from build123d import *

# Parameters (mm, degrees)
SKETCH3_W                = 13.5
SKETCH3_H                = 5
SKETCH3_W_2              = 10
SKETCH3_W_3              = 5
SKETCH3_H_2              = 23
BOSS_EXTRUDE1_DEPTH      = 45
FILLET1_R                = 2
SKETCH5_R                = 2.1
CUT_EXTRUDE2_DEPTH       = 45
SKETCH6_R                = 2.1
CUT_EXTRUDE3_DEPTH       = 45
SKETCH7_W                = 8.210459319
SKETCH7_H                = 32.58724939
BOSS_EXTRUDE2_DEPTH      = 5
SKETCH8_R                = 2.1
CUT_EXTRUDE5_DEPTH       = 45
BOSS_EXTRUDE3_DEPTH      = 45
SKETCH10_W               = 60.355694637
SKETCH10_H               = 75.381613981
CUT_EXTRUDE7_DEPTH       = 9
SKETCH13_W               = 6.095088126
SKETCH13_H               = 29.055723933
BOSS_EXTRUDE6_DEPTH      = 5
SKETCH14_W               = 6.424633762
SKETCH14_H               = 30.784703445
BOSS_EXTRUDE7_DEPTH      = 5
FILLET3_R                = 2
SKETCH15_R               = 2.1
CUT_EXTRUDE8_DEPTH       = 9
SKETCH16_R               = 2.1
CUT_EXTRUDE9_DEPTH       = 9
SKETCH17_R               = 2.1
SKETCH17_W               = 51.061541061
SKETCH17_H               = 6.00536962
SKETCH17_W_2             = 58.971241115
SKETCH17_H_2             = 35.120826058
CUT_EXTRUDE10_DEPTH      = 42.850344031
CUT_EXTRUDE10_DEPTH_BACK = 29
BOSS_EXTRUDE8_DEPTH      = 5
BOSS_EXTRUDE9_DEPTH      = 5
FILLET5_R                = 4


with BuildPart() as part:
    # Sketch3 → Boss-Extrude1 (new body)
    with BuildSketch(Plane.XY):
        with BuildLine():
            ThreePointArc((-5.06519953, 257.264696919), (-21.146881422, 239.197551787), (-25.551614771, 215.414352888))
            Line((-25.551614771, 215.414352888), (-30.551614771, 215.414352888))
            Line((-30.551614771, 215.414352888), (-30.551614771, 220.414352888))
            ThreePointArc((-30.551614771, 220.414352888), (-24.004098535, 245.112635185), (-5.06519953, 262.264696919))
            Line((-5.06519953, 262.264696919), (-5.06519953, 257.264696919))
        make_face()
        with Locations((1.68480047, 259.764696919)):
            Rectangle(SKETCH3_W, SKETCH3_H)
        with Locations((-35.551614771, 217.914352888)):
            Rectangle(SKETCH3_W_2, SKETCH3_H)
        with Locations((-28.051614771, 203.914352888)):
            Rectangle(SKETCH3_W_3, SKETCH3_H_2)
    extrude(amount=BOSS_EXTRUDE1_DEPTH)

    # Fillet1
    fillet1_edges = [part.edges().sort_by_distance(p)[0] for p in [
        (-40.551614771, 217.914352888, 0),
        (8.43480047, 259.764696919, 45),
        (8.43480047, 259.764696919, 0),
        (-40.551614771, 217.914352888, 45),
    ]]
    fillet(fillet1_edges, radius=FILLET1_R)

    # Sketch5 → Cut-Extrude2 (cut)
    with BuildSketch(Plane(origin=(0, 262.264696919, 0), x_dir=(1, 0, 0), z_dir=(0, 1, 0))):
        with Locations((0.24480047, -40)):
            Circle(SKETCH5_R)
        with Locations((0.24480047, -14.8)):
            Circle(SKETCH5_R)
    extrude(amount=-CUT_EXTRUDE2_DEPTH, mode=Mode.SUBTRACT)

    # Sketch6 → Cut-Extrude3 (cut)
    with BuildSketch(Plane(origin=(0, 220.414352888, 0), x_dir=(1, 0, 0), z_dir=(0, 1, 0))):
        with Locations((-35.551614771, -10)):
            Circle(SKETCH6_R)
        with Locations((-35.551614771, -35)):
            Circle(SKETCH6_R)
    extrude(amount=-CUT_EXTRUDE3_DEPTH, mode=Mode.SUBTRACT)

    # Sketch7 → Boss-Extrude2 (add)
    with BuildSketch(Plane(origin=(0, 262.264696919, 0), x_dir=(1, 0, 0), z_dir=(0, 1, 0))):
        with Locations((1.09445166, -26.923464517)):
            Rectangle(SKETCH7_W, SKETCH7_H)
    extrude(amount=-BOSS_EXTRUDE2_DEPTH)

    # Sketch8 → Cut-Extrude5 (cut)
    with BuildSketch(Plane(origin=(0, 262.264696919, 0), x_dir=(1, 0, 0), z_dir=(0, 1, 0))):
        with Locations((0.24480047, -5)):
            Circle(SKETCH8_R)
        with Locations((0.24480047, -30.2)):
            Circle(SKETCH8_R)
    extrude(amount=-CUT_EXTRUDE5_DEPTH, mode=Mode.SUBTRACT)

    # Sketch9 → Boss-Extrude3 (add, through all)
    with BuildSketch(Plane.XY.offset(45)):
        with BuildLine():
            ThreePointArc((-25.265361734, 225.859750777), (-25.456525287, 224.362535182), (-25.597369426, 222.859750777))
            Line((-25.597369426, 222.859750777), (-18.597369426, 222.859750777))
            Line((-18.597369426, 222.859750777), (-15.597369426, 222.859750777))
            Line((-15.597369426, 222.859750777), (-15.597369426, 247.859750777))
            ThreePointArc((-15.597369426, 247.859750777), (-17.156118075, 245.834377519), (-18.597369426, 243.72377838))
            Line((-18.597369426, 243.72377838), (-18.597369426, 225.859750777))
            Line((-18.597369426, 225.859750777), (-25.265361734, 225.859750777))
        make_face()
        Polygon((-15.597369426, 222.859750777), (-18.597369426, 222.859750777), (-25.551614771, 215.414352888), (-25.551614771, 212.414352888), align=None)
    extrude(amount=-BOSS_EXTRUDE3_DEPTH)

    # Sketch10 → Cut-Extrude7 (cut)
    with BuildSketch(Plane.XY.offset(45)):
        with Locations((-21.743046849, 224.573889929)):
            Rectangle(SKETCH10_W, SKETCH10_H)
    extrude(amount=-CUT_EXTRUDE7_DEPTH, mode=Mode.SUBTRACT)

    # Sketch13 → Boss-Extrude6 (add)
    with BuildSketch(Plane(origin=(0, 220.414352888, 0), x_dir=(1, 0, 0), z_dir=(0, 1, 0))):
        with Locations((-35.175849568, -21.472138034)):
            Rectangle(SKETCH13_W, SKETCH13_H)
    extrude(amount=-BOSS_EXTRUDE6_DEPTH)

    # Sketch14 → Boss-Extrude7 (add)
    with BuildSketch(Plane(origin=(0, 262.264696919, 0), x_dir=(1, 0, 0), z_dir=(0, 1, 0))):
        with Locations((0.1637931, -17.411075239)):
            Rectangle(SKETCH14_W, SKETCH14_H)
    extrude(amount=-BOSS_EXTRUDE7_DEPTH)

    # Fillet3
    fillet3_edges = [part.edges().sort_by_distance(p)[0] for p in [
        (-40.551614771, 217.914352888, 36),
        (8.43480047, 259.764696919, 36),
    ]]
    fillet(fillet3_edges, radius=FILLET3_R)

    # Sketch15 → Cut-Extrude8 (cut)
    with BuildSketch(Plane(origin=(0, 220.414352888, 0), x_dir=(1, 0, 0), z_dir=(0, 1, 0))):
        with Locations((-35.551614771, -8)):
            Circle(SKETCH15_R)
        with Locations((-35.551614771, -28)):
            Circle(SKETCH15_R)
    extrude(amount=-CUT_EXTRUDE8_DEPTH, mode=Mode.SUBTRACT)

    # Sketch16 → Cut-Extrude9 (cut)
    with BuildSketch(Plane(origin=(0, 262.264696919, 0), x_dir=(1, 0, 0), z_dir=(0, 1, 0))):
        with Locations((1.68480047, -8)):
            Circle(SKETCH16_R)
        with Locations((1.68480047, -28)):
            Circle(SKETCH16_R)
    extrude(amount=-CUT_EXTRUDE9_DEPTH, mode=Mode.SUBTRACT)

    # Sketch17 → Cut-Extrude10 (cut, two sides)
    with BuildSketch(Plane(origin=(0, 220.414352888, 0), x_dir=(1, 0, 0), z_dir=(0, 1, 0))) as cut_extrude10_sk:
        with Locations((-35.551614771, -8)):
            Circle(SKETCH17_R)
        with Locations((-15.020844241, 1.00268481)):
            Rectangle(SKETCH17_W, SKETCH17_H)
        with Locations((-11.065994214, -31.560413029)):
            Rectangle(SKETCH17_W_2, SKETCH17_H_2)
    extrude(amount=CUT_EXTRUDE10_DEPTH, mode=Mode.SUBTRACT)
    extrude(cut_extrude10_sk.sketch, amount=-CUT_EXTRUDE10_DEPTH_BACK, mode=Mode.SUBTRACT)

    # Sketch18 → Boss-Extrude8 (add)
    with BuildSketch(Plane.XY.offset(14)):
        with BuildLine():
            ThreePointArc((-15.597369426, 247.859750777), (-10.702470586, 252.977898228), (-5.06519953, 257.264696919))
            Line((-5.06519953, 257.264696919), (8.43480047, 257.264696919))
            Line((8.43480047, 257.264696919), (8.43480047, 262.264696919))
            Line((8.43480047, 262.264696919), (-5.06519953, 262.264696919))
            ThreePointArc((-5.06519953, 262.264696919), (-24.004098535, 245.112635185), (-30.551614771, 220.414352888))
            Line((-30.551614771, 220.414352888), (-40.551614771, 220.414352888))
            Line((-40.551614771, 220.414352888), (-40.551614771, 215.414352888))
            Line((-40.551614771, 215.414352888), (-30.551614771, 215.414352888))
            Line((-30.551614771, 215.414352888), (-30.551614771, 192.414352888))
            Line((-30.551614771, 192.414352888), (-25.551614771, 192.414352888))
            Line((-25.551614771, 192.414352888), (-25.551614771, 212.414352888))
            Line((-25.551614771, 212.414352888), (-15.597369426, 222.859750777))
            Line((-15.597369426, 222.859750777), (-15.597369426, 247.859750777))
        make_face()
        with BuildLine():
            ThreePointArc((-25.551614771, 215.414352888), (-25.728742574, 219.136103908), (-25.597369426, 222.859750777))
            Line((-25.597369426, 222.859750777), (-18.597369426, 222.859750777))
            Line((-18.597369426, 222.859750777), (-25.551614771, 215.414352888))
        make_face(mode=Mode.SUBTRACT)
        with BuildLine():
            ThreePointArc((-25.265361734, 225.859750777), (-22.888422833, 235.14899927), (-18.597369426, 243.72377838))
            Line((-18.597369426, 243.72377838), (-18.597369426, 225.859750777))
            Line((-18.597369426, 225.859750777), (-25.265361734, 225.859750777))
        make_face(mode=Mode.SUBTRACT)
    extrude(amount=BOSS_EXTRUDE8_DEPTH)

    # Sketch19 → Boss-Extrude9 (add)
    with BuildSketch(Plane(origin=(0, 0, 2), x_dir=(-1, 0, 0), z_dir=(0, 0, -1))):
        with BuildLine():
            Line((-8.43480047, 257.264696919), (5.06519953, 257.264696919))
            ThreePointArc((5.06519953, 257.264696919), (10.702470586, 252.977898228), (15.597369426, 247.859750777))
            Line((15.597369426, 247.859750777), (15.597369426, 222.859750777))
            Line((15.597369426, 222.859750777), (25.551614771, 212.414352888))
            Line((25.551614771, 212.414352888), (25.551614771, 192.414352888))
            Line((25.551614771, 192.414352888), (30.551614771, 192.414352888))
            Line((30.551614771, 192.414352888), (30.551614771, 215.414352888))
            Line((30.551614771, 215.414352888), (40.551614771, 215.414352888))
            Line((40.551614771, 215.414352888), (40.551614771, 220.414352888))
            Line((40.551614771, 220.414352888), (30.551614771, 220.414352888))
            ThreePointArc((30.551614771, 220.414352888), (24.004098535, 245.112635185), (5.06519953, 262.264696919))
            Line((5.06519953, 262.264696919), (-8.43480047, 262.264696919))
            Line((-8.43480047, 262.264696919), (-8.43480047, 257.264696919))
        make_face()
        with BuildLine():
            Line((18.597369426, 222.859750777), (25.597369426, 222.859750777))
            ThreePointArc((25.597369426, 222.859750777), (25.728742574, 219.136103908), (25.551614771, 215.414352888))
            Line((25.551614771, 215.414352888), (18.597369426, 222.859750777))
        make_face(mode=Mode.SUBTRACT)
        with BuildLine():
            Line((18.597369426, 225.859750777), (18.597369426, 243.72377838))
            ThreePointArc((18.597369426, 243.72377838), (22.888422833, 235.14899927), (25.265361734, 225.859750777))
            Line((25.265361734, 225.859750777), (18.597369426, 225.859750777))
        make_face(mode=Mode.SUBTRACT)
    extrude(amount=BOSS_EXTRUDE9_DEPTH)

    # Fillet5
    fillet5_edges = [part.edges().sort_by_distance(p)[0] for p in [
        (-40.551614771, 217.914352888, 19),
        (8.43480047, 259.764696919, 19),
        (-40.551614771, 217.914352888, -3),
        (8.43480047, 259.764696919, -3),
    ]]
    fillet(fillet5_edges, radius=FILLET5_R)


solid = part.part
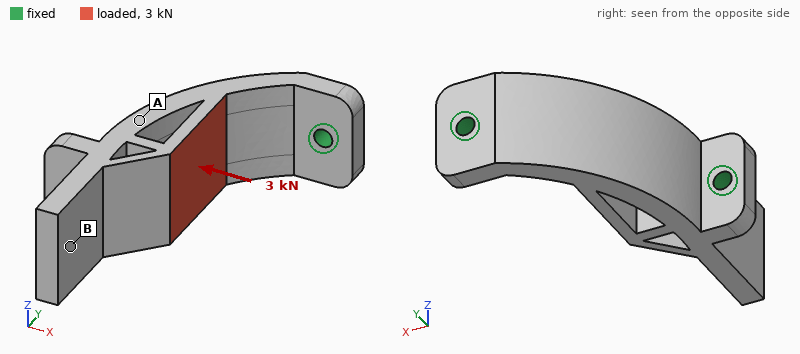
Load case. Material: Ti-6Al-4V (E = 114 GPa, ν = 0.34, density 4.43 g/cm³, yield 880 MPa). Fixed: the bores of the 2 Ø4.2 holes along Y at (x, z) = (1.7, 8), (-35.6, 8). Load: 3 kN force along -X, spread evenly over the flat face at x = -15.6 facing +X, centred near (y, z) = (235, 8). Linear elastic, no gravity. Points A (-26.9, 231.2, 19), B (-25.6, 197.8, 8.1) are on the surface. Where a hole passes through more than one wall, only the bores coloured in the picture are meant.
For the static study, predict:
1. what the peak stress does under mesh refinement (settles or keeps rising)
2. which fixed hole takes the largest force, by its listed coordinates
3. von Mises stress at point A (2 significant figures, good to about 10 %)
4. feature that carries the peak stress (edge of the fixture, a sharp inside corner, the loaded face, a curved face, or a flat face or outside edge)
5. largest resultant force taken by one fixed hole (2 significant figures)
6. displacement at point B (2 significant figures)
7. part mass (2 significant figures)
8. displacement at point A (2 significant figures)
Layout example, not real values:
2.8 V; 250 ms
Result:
keeps rising; (1.7, 8); 18 MPa; edge of the fixture; 2.0 kN; 17 µm; 59 g; 18 µm
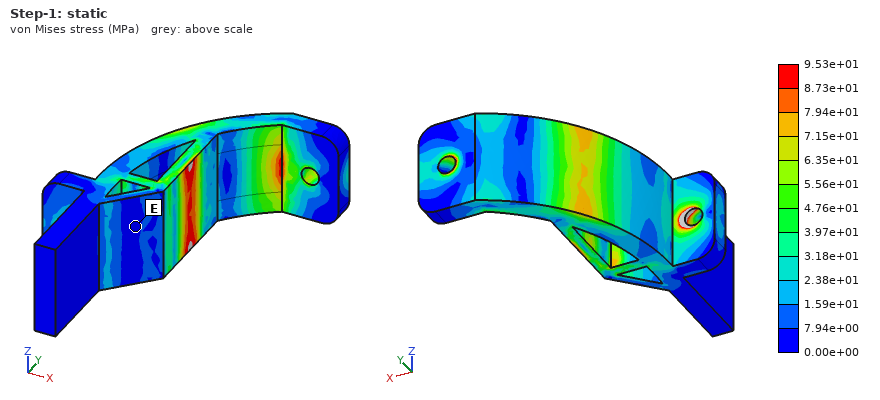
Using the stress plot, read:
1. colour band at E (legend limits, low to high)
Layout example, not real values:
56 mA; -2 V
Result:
0.00e+00 to 7.94e+00 MPa
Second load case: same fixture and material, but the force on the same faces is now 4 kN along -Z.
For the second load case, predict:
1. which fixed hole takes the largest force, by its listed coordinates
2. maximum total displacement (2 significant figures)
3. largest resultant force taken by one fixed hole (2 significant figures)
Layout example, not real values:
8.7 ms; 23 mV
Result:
(-35.6, 8); 61 µm; 2.3 kN
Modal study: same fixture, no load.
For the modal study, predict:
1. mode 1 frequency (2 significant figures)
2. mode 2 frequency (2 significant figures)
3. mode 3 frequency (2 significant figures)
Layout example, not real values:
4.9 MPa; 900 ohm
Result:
6100 Hz; 6800 Hz; 9500 Hz
